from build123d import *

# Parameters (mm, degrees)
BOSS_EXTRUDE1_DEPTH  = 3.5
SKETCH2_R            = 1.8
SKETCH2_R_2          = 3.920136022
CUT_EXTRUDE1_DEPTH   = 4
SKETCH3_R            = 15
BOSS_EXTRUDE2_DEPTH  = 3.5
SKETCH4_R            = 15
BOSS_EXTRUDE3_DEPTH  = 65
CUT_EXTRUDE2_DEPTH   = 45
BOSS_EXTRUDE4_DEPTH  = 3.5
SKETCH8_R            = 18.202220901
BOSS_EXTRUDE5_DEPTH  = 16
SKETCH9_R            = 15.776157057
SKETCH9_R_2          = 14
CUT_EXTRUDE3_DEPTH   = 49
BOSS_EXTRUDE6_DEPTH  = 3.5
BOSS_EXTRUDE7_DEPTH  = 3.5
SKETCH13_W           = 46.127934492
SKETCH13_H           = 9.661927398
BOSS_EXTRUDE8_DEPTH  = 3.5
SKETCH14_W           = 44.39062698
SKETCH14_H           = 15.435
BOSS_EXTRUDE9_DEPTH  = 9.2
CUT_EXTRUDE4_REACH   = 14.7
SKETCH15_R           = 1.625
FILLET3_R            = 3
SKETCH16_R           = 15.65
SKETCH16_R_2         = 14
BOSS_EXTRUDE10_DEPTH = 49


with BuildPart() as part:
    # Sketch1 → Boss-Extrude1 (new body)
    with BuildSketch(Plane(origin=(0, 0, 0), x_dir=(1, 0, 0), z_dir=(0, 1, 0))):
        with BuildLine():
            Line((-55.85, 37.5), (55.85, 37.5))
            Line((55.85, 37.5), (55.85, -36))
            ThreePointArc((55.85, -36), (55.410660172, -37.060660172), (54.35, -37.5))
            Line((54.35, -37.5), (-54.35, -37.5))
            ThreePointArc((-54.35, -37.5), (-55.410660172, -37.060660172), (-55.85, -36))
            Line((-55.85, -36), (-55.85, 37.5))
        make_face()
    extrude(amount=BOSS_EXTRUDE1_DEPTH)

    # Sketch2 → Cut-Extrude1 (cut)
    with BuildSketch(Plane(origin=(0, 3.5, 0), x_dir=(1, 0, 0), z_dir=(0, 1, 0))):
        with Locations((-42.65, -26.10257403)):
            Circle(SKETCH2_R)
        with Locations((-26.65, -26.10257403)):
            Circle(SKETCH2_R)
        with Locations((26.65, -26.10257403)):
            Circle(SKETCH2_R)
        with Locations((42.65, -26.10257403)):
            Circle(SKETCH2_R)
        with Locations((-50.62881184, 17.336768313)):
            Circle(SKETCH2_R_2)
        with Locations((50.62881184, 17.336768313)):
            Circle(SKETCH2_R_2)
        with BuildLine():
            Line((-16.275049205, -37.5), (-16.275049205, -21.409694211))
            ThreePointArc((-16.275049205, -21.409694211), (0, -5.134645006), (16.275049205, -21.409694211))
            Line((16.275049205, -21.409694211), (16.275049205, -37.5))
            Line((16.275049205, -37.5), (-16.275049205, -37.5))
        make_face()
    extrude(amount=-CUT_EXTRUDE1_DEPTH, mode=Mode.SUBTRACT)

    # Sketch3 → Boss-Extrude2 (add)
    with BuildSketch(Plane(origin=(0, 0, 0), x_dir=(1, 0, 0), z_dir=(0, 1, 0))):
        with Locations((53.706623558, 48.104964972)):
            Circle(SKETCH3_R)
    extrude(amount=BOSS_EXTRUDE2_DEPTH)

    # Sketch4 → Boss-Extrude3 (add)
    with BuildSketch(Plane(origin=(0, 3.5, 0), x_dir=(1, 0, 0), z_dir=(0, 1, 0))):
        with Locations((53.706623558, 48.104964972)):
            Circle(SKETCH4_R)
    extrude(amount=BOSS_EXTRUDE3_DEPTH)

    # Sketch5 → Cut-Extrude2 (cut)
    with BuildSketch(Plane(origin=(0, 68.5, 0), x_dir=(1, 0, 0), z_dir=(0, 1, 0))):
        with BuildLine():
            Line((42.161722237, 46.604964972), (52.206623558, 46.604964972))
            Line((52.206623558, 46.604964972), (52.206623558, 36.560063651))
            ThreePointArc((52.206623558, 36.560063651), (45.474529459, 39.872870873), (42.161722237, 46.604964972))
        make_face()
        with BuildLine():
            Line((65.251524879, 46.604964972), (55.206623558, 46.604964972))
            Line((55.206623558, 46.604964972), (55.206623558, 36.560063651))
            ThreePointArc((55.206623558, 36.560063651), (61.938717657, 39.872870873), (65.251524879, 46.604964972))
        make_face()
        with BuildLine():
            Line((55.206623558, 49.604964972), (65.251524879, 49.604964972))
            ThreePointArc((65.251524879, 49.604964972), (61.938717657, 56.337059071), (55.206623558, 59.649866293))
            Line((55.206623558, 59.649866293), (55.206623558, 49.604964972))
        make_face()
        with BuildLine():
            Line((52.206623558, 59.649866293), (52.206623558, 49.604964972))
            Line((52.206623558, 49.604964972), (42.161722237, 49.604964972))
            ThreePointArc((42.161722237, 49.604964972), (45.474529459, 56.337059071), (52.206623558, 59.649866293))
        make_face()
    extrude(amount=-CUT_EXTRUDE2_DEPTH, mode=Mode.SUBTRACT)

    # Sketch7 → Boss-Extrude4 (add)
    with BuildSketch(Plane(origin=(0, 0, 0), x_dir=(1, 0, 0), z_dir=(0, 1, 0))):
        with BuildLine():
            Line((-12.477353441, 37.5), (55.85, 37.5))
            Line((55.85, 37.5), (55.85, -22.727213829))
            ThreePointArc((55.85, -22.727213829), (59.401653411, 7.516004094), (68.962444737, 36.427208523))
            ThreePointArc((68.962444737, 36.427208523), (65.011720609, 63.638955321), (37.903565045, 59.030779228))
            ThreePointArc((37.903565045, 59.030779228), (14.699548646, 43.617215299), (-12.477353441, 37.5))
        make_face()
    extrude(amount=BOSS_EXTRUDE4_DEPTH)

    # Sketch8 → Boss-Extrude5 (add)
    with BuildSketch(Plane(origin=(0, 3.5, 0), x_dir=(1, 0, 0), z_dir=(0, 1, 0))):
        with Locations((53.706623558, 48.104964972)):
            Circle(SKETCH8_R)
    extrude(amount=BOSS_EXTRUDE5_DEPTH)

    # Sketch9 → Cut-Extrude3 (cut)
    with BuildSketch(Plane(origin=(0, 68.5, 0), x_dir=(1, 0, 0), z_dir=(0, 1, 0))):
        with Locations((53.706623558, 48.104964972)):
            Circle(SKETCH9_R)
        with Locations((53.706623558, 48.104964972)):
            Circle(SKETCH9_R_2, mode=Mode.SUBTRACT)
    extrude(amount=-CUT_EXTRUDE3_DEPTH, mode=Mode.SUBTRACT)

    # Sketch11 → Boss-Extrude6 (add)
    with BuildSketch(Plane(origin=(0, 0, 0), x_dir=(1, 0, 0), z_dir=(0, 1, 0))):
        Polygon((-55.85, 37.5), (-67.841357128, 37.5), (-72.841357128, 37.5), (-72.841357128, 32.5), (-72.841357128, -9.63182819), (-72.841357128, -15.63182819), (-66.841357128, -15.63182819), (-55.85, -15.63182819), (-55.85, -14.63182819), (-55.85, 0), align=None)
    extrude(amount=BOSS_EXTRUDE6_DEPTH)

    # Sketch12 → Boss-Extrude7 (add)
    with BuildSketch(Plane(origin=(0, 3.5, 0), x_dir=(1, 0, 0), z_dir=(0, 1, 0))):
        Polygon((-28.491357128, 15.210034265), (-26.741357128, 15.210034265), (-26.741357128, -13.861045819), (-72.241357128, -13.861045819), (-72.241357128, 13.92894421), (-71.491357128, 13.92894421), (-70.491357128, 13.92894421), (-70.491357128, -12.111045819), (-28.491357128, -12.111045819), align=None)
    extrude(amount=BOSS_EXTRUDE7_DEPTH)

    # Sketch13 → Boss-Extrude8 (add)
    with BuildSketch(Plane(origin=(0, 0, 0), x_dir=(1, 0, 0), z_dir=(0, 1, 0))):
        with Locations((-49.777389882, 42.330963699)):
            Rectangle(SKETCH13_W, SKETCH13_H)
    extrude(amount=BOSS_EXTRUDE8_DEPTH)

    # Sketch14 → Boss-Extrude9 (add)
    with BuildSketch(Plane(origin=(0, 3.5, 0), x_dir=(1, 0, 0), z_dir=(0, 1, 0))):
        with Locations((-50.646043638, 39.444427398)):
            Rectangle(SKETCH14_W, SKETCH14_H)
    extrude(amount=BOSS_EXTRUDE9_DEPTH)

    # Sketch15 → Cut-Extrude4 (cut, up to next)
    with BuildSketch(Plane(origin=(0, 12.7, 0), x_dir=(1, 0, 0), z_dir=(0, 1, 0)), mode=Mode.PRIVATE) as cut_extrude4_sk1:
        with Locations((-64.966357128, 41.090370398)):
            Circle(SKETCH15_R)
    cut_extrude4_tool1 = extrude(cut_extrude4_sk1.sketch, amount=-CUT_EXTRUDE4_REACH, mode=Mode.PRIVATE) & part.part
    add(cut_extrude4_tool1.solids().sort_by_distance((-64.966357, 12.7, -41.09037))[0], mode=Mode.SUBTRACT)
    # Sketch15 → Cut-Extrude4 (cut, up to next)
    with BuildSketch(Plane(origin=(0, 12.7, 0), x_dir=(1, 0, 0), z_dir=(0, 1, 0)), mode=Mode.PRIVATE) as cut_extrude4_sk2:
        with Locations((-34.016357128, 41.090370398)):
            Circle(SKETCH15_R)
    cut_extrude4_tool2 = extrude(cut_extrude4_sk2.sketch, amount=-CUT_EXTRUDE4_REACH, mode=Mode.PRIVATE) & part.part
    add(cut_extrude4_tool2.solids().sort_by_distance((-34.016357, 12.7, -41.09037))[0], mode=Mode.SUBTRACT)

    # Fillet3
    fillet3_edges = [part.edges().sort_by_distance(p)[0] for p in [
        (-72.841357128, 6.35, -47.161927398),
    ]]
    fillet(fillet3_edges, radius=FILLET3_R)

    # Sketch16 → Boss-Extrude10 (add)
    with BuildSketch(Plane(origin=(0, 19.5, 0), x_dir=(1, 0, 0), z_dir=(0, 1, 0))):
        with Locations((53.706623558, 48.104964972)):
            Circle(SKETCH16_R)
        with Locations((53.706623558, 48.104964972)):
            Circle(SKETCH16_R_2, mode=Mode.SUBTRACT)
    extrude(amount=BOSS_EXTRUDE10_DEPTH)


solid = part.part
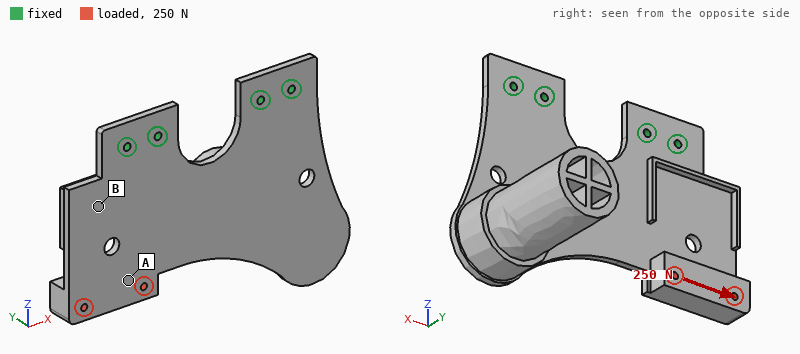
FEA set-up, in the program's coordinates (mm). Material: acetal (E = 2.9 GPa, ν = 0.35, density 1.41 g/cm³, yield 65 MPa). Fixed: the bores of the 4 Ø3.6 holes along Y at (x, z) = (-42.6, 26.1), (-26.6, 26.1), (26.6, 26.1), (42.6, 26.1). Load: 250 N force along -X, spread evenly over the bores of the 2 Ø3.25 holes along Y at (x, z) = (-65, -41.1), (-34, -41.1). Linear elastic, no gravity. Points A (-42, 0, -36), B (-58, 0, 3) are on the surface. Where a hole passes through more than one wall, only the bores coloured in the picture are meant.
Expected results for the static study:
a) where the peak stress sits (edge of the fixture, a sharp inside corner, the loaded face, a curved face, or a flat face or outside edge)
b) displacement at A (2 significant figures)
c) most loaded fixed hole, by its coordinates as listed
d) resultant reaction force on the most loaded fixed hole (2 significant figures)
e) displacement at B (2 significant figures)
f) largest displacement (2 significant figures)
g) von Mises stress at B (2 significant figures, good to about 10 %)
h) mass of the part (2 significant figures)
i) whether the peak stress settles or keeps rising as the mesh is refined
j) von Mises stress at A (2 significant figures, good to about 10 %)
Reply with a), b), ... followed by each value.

a) edge of the fixture
b) 0.66 mm
c) (-42.6, 26.1)
d) 230 N
e) 0.53 mm
f) 2.2 mm
g) 5.3 MPa
h) 120 g
i) keeps rising
j) 1.4 MPa
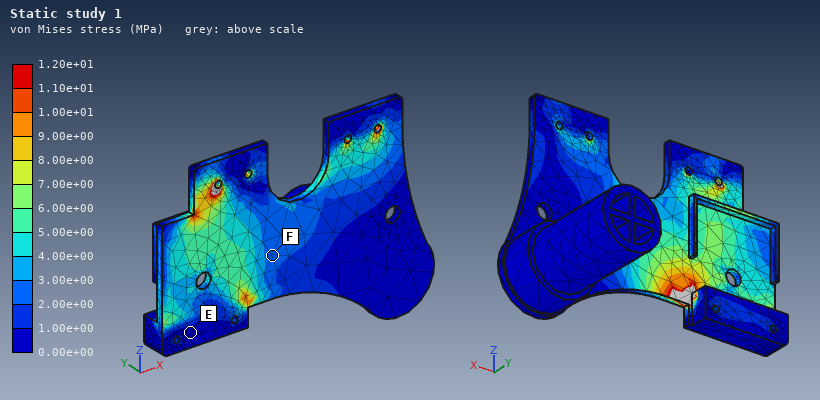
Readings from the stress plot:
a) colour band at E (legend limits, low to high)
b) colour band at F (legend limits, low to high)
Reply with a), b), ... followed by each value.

a) 0.00e+00 to 1.00e+00 MPa
b) 2.00e+00 to 3.00e+00 MPa
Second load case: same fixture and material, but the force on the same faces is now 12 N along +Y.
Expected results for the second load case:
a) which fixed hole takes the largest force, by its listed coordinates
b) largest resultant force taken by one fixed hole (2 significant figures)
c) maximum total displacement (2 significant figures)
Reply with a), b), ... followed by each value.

a) (-42.6, 26.1)
b) 12 N
c) 2.2 mm
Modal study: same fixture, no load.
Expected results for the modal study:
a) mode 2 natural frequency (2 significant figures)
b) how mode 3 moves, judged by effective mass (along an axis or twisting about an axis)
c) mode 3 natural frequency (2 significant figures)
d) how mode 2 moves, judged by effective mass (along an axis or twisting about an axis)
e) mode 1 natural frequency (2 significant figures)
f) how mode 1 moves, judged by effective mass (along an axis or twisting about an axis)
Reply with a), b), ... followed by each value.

a) 78 Hz
b) along Y
c) 130 Hz
d) along X
e) 35 Hz
f) along Y
